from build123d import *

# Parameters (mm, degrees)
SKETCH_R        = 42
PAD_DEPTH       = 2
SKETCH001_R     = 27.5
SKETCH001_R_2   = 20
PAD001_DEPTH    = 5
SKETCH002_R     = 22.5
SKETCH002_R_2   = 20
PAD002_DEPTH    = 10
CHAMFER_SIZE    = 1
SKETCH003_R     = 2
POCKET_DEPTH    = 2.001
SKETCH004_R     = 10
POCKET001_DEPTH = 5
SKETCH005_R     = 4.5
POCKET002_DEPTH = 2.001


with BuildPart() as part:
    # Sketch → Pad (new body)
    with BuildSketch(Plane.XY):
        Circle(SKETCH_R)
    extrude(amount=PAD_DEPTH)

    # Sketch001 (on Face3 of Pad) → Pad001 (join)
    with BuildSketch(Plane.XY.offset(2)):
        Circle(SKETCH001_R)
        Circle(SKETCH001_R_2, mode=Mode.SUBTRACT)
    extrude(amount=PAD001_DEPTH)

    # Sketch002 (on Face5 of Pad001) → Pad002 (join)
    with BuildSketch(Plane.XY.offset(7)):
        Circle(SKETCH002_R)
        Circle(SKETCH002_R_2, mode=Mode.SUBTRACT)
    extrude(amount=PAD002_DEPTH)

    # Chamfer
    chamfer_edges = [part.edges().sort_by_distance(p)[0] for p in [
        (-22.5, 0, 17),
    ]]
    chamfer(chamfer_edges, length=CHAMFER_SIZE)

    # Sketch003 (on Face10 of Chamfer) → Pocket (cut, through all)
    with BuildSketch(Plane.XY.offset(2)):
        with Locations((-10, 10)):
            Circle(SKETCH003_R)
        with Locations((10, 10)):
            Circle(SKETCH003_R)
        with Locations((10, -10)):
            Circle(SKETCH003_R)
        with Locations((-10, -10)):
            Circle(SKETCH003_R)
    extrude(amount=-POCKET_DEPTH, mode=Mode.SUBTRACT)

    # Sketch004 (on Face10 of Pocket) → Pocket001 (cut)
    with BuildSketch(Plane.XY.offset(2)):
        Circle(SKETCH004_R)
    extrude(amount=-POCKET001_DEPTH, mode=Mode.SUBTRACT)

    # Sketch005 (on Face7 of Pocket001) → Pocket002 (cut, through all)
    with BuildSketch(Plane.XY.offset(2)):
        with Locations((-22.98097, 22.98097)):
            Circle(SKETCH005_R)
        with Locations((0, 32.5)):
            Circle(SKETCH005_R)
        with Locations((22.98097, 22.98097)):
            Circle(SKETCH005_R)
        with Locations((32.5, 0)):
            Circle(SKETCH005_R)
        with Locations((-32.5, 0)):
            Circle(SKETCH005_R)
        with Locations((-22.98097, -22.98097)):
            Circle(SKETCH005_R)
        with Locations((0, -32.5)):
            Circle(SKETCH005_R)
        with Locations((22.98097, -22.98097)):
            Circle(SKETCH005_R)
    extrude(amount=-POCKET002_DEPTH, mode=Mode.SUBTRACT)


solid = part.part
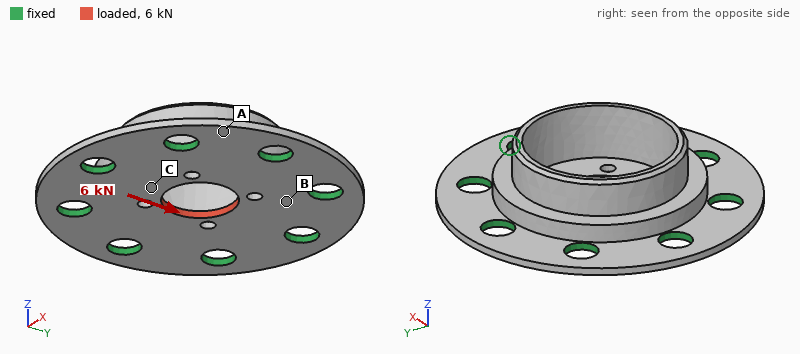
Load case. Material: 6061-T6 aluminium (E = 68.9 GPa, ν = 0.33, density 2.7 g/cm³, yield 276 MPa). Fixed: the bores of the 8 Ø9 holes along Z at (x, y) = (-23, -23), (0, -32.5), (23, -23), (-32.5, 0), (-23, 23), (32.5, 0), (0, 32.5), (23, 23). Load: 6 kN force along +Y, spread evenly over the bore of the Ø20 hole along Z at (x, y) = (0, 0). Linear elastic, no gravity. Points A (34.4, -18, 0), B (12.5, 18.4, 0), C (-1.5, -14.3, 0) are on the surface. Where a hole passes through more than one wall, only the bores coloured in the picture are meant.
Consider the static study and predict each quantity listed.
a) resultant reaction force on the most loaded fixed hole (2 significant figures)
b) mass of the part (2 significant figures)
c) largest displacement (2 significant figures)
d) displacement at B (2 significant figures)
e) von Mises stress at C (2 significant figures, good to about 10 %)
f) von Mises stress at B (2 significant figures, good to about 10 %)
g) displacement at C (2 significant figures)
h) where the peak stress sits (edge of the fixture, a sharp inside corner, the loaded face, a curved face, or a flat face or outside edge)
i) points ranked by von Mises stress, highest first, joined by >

1.2 kN
49 g
15 µm
3.3 µm
42 MPa
27 MPa
9.4 µm
a curved face
C > B > A
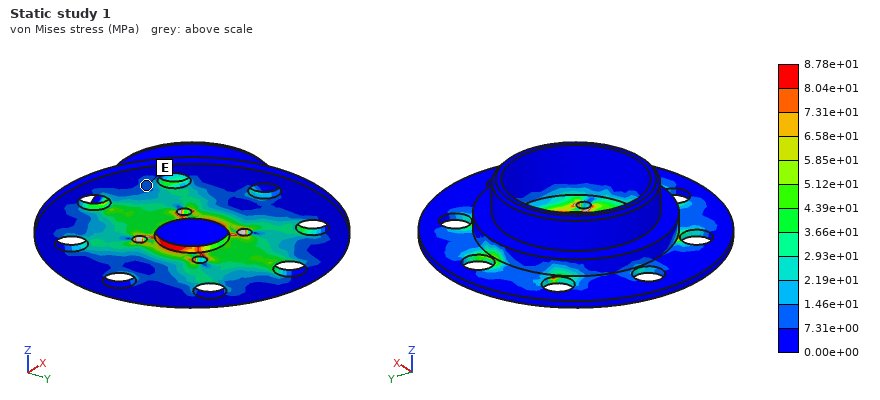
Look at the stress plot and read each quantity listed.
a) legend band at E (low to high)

7.31e+00 to 1.46e+01 MPa
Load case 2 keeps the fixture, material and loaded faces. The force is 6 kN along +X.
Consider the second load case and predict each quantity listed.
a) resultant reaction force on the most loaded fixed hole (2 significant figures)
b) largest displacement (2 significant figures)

1.2 kN
15 µm
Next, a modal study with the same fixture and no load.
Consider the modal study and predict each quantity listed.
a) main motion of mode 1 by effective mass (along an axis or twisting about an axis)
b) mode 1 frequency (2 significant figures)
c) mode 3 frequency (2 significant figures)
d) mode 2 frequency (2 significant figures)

along Z
14 kHz
18 kHz
18 kHz
